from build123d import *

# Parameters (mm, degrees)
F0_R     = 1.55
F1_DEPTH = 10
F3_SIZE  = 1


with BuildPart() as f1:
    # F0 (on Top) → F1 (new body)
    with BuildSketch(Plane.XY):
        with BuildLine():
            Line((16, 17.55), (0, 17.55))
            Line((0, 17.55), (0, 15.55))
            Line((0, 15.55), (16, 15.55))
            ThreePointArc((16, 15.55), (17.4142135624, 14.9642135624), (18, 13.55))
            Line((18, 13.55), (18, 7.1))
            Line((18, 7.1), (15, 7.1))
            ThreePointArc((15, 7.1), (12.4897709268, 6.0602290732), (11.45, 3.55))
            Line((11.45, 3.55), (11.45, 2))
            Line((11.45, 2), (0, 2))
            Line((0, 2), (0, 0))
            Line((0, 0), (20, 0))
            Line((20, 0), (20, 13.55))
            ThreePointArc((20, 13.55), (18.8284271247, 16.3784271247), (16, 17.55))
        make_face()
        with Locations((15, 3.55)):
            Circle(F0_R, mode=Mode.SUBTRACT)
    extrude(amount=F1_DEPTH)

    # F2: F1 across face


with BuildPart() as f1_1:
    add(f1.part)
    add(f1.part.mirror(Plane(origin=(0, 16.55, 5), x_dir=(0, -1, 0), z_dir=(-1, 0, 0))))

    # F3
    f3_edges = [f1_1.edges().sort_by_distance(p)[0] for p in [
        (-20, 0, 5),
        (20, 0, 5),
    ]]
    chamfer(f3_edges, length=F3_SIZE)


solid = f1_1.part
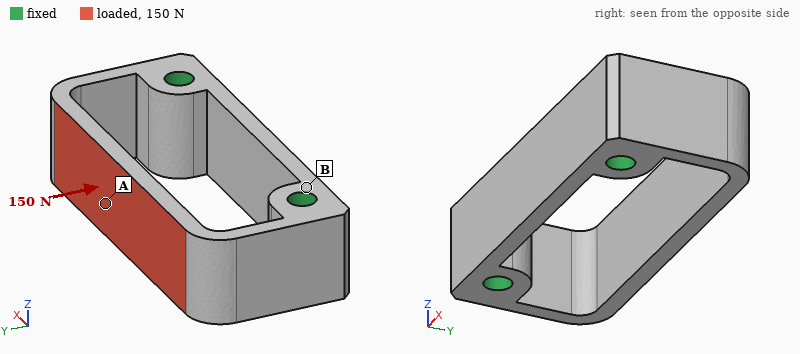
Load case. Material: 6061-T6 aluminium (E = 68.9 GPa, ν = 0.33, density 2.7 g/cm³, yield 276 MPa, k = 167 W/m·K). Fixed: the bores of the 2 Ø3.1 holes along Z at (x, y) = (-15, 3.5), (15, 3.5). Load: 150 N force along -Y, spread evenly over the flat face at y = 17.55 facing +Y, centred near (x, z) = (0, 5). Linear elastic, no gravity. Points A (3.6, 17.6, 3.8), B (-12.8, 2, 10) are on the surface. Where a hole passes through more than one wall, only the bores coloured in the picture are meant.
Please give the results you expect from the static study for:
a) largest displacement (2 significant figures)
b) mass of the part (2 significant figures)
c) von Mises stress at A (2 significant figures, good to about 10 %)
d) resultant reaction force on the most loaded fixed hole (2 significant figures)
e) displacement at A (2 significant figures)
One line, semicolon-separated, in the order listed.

71 µm; 6.9 g; 44 MPa; 110 N; 64 µm
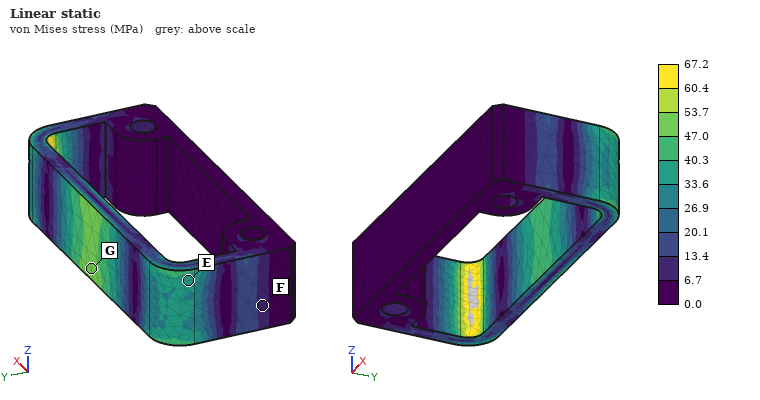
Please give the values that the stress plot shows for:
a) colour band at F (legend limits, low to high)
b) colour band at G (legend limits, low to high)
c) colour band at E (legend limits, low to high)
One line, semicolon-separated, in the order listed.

6.7 to 13.4 MPa; 47.0 to 53.7 MPa; 33.6 to 40.3 MPa
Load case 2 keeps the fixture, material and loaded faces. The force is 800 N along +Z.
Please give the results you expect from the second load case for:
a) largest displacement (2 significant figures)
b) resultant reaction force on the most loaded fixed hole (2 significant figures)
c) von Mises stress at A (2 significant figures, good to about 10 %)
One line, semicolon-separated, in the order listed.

0.12 mm; 400 N; 33 MPa
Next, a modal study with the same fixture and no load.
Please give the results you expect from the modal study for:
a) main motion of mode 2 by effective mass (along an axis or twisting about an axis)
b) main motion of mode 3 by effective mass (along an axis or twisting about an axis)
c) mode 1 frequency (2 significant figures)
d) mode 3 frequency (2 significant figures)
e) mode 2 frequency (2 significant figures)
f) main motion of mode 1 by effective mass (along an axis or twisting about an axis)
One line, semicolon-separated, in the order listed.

along X; along Z; 6400 Hz; 11 kHz; 7000 Hz; along Y
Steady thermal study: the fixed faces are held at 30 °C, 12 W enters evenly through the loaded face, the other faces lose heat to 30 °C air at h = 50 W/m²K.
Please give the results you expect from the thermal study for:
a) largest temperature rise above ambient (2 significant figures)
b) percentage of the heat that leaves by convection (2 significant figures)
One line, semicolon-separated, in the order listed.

36 K; 8.8 %
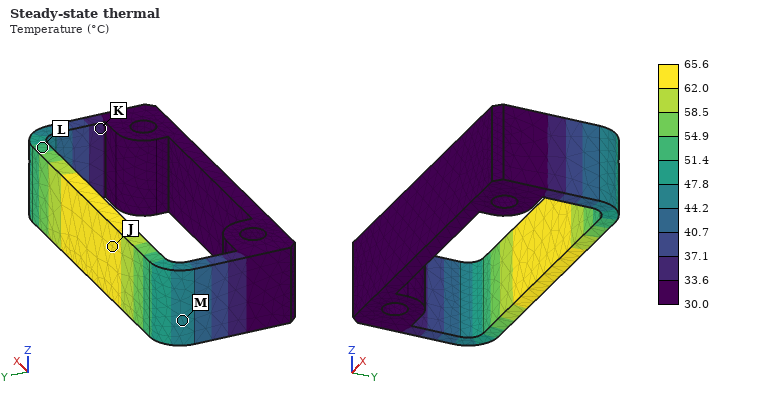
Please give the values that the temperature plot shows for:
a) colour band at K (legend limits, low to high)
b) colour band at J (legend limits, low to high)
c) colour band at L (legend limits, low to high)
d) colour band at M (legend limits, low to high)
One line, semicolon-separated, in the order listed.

33.6 to 37.1 °C; 62.0 to 65.6 °C; 51.4 to 54.9 °C; 44.2 to 47.8 °C
